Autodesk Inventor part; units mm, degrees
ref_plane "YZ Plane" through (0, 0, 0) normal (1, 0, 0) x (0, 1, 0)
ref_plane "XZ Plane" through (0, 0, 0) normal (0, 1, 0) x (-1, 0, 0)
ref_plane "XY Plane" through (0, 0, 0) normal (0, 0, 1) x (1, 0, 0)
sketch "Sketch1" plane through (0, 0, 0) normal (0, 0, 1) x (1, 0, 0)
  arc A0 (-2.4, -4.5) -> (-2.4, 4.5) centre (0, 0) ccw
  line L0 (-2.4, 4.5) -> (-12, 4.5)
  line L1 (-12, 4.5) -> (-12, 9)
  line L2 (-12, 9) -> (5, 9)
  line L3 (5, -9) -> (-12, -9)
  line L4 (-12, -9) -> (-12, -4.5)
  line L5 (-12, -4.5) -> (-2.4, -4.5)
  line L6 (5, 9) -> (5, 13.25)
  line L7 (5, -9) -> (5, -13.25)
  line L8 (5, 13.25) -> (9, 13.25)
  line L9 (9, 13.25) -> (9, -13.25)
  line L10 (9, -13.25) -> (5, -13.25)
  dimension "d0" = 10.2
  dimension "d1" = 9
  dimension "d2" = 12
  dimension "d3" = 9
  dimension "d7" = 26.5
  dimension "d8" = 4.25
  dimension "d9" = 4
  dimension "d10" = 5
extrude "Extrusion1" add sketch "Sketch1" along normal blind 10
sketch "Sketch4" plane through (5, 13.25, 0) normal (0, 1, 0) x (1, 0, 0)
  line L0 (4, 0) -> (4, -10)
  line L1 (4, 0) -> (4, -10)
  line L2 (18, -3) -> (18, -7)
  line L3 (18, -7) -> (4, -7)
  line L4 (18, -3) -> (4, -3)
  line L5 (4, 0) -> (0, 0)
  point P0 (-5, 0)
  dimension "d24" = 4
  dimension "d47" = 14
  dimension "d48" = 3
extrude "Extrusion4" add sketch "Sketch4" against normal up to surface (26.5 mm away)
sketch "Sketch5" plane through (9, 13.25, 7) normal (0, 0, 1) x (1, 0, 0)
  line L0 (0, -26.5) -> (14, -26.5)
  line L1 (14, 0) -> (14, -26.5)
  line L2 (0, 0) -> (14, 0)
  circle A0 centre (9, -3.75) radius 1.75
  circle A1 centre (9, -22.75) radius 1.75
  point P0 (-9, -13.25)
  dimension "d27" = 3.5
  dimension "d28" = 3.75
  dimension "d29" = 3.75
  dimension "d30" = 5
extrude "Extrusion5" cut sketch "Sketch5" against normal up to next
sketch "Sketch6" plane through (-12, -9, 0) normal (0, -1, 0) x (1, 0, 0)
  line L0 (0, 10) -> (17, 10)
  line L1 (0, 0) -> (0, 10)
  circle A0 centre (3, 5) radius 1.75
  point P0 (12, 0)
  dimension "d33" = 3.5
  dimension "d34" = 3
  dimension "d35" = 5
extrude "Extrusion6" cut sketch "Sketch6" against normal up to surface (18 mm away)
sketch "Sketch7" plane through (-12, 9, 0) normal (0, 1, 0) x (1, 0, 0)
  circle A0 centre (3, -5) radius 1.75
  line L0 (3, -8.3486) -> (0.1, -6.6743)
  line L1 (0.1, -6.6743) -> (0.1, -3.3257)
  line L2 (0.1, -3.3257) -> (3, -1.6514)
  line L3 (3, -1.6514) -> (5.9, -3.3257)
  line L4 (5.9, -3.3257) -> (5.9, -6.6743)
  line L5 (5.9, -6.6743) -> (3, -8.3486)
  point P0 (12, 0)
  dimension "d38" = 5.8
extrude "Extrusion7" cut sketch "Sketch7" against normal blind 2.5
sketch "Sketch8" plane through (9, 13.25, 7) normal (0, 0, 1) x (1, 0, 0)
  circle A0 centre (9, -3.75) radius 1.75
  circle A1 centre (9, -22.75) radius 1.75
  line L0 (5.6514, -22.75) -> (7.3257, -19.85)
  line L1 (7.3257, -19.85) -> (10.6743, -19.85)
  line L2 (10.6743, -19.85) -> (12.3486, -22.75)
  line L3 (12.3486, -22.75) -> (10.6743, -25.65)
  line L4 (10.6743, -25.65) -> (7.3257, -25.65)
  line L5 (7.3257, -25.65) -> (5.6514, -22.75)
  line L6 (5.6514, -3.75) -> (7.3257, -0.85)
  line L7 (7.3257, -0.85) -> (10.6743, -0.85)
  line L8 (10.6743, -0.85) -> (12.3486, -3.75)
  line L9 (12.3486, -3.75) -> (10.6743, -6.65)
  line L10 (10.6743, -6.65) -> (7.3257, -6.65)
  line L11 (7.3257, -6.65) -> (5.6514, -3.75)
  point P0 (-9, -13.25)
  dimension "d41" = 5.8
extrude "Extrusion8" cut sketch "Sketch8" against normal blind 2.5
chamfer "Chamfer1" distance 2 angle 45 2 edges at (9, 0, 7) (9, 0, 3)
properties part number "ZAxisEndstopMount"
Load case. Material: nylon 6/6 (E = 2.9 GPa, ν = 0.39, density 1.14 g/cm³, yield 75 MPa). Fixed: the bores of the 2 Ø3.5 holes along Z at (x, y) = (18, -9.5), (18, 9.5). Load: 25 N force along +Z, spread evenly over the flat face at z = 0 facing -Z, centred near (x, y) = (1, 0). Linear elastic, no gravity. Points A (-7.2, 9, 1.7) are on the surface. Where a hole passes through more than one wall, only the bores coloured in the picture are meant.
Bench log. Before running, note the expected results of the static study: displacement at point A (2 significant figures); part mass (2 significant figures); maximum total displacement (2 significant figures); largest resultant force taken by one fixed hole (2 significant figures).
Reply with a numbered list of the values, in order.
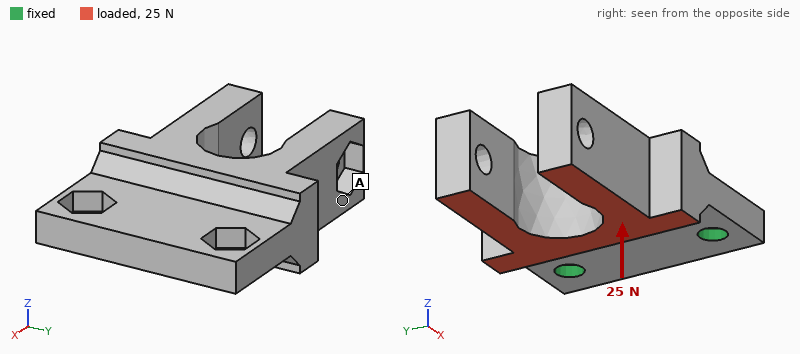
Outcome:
1. 0.38 mm
2. 4.4 g
3. 0.47 mm
4. 13 N
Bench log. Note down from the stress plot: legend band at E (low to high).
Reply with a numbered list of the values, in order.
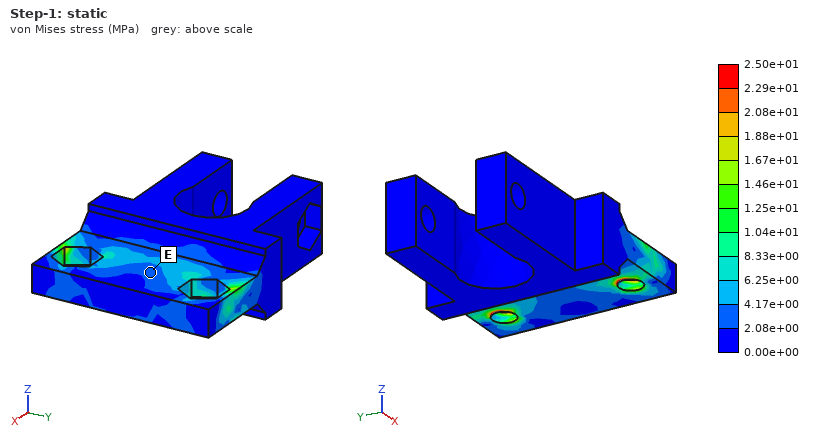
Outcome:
1. 2.08e+00 to 4.17e+00 MPa
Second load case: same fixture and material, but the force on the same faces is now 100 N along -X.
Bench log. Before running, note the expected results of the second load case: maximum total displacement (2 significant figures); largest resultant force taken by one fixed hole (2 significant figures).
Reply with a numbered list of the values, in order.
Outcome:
1. 0.52 mm
2. 51 N
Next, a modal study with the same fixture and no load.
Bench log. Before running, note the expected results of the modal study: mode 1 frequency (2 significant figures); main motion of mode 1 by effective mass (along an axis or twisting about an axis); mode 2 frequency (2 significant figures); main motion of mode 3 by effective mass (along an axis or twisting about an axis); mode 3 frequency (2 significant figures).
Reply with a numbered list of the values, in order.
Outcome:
1. 880 Hz
2. along Z
3. 2900 Hz
4. along Y
5. 3400 Hz
